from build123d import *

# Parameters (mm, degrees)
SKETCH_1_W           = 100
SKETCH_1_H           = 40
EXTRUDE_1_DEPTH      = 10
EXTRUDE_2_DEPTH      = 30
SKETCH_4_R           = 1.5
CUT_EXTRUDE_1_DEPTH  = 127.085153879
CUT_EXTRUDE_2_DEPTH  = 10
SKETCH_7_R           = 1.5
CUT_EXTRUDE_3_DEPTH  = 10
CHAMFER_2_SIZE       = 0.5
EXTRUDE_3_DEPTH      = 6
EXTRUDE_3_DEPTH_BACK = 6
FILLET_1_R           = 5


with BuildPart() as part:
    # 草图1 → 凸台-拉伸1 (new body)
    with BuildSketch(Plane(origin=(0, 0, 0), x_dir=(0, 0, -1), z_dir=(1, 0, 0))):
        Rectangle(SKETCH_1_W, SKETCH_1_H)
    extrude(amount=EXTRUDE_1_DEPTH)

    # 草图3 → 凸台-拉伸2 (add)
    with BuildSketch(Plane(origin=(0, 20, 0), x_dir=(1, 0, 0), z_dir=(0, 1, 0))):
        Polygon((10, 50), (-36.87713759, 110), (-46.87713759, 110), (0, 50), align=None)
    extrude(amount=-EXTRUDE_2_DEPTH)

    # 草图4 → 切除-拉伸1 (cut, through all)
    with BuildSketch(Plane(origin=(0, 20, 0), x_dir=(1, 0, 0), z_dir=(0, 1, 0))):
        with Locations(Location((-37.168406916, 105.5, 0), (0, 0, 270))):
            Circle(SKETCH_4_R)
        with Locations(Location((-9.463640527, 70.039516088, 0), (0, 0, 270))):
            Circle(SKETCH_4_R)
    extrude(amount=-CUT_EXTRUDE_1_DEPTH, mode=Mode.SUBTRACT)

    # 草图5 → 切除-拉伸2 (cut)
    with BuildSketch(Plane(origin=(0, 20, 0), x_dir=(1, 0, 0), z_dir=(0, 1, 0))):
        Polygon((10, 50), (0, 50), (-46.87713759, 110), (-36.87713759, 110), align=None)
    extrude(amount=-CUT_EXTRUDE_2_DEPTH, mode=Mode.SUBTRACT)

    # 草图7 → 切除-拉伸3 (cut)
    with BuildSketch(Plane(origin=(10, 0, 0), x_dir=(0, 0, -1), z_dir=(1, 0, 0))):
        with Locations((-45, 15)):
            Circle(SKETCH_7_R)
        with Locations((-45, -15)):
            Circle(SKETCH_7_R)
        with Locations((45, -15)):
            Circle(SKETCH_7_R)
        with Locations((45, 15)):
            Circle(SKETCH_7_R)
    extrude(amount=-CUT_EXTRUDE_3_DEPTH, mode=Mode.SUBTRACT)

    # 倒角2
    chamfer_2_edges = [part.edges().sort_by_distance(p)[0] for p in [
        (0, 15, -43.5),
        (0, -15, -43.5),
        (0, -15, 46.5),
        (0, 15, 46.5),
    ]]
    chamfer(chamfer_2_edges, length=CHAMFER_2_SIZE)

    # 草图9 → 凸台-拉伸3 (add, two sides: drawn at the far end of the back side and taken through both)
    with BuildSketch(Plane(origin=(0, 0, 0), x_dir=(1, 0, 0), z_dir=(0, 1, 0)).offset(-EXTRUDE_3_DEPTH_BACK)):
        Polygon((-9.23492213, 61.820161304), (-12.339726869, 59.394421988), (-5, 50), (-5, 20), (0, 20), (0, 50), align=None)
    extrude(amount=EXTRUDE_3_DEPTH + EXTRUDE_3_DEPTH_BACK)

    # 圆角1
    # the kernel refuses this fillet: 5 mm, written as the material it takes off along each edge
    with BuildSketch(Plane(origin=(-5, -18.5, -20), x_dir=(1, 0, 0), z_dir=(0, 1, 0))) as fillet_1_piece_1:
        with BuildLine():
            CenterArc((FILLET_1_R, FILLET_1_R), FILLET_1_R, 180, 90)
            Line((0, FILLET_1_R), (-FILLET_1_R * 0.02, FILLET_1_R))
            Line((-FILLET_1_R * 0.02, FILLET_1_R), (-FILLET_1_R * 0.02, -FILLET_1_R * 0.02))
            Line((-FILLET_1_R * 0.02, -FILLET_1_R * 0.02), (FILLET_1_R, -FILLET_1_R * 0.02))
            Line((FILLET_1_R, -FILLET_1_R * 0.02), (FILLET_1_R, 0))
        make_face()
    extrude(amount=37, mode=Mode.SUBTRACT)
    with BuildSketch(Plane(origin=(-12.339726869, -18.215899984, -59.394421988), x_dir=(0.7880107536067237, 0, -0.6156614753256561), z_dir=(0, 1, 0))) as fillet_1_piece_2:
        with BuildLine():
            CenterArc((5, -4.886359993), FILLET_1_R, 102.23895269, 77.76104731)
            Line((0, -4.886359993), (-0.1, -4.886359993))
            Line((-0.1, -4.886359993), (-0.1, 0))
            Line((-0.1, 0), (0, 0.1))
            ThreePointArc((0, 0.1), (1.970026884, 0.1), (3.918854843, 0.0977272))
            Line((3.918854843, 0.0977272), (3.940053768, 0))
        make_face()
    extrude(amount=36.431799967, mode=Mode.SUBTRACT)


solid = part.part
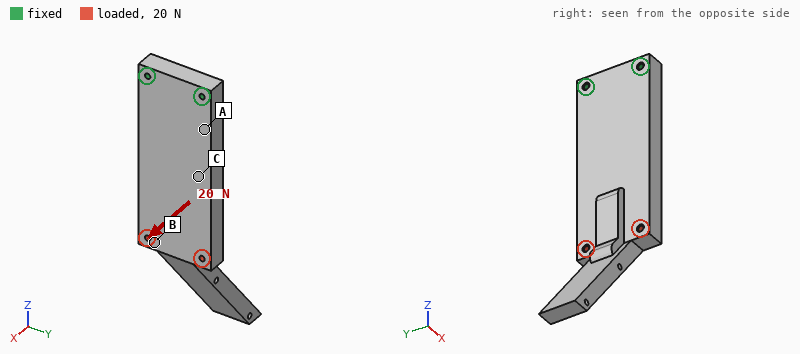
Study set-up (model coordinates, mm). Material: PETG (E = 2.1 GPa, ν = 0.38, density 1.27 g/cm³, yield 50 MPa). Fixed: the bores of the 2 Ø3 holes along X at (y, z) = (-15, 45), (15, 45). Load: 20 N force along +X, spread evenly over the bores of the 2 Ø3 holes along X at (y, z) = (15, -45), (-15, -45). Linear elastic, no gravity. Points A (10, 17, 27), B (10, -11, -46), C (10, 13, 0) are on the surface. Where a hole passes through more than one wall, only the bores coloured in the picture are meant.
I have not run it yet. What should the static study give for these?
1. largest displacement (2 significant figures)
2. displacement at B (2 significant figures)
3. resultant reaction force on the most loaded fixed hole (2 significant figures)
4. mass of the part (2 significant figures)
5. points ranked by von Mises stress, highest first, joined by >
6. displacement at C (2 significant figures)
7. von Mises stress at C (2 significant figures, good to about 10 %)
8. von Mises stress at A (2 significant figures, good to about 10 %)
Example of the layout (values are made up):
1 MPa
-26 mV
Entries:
1.8 mm
0.83 mm
10 N
68 g
A > C > B
0.29 mm
1.4 MPa
2.3 MPa
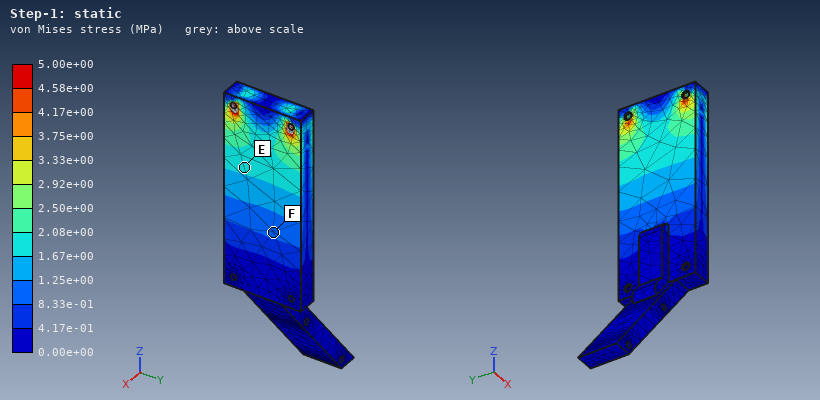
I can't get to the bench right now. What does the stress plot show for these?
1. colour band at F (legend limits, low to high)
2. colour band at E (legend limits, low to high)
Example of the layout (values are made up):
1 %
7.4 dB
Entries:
8.33e-01 to 1.25e+00 MPa
1.67e+00 to 2.08e+00 MPa
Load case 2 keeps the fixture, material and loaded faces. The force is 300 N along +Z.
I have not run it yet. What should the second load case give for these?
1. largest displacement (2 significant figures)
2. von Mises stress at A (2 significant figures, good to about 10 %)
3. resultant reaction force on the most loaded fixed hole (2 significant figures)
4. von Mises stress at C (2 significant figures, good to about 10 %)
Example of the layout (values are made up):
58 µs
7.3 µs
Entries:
0.14 mm
0.99 MPa
150 N
0.86 MPa
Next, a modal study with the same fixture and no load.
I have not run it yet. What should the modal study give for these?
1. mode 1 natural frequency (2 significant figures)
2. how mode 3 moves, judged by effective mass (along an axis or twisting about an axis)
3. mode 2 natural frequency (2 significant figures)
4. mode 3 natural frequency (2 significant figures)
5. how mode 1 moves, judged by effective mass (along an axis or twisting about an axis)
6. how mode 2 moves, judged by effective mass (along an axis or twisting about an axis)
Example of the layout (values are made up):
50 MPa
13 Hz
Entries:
100 Hz
along X
300 Hz
400 Hz
along X
along Y
